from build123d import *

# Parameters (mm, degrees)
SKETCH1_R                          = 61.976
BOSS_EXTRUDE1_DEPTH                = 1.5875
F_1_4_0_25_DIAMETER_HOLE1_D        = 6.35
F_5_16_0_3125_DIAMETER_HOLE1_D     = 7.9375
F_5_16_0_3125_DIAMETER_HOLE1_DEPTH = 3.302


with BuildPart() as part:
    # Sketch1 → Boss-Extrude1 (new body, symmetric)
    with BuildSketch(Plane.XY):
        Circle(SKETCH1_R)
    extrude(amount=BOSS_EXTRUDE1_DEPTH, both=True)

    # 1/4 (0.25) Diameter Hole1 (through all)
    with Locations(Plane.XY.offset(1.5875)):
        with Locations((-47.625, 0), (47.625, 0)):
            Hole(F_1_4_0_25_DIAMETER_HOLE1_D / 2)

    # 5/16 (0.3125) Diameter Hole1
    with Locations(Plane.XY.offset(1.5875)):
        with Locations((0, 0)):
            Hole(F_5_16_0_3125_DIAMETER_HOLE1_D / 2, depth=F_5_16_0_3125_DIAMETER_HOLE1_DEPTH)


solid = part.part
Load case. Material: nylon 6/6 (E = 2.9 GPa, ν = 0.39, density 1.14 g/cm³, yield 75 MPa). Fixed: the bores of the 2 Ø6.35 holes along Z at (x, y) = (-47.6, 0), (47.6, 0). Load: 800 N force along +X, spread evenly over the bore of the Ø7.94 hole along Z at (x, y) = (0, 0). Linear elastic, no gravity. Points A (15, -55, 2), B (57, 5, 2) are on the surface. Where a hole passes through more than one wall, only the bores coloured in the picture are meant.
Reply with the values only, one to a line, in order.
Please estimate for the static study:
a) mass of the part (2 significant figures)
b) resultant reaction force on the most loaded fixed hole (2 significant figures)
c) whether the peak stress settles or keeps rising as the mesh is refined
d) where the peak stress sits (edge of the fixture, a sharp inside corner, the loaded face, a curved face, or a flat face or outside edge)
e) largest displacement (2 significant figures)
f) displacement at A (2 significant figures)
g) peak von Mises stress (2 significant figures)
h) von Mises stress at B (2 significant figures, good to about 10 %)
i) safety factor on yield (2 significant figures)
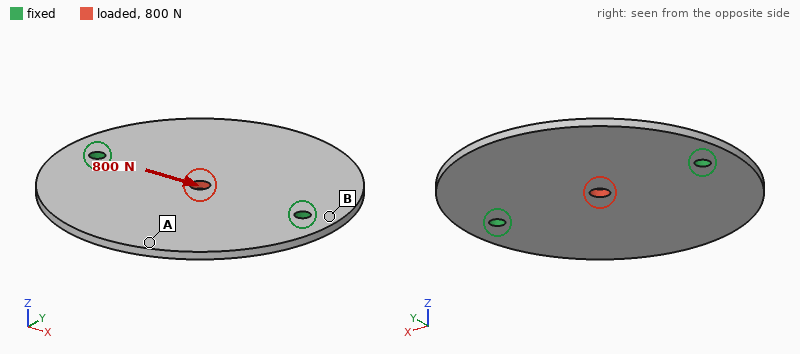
43 g
400 N
settles
the loaded face
86 µm
32 µm
17 MPa
2.1 MPa
4.3
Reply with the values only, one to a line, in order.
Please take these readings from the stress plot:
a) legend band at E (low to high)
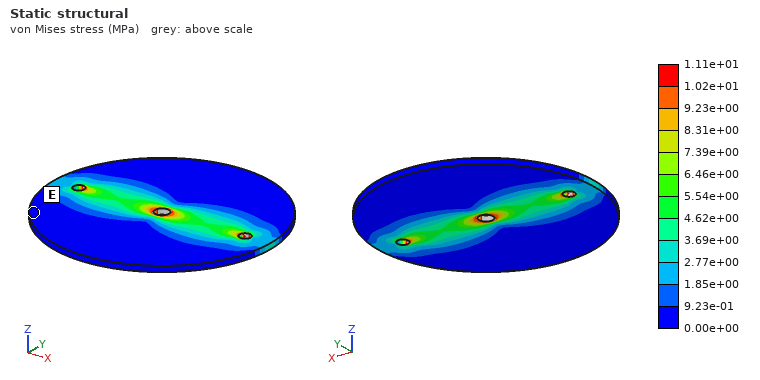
0.00e+00 to 9.23e-01 MPa
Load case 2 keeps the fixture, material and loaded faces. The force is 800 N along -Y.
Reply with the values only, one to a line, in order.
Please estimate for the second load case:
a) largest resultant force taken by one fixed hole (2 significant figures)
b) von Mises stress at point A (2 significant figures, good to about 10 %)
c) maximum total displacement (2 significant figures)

400 N
1.8 MPa
0.12 mm
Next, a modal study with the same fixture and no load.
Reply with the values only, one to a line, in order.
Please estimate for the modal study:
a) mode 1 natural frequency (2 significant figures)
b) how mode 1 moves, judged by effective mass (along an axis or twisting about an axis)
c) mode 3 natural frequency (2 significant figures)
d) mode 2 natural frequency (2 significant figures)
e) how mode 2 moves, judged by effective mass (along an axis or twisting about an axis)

200 Hz
twisting about X
550 Hz
260 Hz
along Z
